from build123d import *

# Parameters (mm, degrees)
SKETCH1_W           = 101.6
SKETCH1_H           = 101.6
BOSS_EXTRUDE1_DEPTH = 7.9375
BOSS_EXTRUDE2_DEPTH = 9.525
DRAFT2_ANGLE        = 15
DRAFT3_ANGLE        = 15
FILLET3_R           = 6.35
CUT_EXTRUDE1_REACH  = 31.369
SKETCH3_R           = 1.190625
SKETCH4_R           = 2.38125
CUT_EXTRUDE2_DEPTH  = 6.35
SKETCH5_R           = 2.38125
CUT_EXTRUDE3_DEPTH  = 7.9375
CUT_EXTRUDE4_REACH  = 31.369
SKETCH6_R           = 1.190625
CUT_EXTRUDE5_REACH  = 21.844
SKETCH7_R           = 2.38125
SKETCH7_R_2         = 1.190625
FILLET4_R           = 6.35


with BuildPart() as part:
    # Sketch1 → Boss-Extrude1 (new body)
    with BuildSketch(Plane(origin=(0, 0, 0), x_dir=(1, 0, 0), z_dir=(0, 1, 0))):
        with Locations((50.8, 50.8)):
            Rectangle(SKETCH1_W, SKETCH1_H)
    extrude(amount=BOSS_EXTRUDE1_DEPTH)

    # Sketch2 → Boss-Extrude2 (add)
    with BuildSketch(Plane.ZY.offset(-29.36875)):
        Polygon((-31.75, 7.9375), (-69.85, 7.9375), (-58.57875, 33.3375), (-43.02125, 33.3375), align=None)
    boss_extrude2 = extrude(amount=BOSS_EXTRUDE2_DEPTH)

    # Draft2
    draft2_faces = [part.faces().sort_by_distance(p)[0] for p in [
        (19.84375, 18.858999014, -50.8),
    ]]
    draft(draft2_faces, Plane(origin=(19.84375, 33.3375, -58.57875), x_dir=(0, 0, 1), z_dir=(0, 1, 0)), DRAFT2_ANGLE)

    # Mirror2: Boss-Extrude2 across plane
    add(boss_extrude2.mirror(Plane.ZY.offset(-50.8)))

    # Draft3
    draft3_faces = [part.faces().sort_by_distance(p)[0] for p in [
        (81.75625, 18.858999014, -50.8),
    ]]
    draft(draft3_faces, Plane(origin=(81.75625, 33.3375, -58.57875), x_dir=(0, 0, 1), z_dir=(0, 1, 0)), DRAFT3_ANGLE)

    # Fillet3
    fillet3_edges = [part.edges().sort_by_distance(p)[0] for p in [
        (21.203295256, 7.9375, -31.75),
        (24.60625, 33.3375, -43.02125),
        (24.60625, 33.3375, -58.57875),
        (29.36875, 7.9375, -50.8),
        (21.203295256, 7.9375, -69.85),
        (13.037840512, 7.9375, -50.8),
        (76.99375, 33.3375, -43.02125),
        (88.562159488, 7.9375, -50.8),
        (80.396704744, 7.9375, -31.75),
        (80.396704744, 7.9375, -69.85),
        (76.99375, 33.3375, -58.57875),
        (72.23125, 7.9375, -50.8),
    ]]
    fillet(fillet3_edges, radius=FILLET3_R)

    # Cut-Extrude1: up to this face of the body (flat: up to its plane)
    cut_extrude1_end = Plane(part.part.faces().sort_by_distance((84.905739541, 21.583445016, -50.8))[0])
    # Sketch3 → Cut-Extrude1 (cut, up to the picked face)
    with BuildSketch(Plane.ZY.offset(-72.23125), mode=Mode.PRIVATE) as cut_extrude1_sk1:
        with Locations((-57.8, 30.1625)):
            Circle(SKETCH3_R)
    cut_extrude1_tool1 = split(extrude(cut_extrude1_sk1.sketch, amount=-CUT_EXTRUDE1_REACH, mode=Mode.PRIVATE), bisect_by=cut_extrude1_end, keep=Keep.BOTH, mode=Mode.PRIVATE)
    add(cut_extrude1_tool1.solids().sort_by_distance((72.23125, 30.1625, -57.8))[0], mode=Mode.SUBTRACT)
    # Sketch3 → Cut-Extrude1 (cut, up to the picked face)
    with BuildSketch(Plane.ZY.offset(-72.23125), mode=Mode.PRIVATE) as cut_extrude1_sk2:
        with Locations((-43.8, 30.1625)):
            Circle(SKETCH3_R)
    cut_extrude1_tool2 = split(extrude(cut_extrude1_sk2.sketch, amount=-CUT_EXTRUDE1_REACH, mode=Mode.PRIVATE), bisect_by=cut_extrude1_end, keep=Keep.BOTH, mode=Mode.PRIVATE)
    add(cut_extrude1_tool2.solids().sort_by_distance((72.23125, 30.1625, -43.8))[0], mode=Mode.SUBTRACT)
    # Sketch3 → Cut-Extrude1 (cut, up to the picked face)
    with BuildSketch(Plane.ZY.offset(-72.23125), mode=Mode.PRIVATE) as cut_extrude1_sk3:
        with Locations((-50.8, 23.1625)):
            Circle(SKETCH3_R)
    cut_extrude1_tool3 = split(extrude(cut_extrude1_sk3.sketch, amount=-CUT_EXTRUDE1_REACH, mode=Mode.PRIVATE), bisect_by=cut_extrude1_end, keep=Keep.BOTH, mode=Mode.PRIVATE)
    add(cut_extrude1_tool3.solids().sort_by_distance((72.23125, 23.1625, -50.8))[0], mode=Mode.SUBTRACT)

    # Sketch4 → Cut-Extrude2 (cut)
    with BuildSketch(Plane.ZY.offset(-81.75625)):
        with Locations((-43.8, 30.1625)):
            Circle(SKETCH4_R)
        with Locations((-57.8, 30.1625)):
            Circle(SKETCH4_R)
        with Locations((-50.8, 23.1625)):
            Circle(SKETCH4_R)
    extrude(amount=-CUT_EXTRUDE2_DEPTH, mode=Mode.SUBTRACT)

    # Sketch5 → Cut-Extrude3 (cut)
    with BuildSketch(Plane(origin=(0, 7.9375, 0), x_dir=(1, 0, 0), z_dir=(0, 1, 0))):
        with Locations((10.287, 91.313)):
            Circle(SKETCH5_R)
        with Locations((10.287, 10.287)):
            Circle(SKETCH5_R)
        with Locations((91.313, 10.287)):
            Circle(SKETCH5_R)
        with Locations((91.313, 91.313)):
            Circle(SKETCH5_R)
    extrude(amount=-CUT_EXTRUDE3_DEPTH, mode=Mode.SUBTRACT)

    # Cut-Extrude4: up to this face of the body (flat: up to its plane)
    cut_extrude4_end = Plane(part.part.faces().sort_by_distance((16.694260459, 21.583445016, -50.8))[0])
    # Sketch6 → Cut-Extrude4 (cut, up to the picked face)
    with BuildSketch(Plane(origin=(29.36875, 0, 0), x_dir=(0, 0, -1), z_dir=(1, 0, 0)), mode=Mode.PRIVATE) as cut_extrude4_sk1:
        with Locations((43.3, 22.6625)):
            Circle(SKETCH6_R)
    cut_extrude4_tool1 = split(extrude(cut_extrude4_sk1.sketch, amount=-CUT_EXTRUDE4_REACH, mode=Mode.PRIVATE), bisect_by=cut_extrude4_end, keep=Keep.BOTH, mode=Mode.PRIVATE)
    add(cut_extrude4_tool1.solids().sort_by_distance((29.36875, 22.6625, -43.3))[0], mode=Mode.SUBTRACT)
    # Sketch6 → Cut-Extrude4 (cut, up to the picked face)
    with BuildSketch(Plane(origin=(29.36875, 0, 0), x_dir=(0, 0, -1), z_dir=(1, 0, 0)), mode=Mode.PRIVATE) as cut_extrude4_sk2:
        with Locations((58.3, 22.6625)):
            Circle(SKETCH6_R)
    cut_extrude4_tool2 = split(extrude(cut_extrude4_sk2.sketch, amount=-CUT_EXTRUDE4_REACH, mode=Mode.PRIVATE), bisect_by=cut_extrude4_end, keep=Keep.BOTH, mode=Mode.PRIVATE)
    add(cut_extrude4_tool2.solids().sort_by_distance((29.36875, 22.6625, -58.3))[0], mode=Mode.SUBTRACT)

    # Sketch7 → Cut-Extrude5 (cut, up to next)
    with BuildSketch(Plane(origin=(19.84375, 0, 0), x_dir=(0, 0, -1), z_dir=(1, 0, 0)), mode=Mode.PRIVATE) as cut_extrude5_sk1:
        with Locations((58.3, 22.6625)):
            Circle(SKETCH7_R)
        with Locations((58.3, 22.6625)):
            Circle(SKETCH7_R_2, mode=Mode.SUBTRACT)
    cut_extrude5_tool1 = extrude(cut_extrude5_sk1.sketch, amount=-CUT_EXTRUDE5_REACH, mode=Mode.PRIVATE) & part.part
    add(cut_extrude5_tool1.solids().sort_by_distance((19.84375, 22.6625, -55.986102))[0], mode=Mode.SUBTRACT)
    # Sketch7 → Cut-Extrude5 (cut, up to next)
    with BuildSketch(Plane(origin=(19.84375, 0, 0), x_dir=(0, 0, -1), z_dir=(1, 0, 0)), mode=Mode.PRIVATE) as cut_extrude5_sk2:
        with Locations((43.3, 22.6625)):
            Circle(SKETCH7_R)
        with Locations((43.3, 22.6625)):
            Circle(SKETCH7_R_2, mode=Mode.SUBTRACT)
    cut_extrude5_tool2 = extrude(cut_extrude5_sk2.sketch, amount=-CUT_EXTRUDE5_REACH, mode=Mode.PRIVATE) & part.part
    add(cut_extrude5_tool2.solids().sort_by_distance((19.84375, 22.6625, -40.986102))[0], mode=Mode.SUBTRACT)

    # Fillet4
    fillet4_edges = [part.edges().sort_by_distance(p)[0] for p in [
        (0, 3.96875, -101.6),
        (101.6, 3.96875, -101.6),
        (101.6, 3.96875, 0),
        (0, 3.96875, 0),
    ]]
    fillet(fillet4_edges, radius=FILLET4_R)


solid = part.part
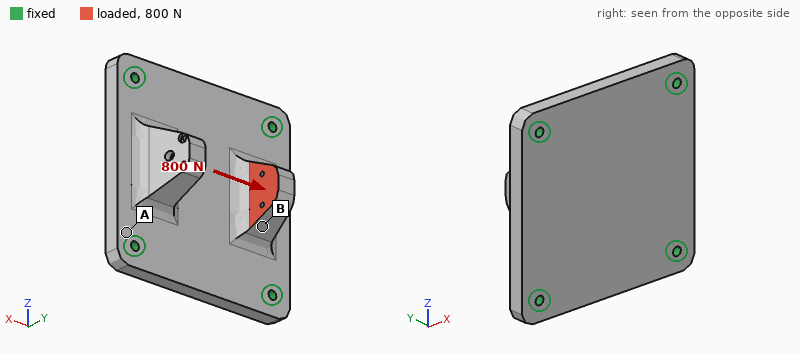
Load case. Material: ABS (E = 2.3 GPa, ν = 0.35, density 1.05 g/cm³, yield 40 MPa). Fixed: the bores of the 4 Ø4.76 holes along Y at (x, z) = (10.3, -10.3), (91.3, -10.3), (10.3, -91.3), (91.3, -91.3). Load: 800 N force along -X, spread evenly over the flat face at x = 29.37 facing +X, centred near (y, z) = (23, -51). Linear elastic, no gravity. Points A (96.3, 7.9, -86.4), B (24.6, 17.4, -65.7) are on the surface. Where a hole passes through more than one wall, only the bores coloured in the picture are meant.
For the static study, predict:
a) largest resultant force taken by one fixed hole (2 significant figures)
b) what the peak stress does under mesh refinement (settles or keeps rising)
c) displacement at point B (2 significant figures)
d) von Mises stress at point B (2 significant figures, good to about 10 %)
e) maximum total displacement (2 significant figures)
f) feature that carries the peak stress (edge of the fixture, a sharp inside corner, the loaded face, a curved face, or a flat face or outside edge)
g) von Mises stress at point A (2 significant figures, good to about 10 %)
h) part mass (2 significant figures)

270 N
keeps rising
0.27 mm
5.1 MPa
0.67 mm
edge of the fixture
1.5 MPa
110 g
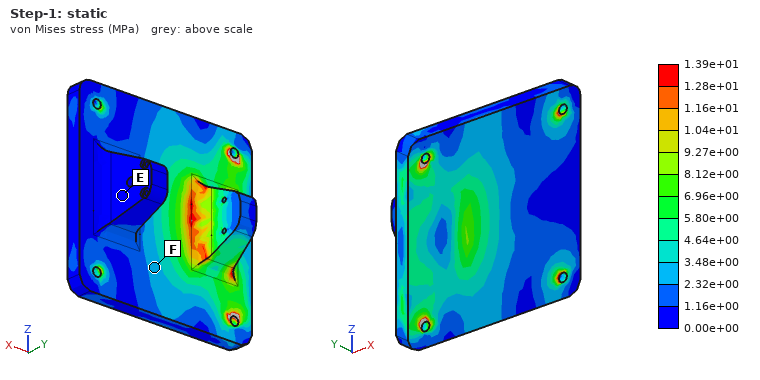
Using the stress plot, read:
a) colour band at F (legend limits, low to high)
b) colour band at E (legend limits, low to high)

2.32e+00 to 3.48e+00 MPa
0.00e+00 to 1.16e+00 MPa
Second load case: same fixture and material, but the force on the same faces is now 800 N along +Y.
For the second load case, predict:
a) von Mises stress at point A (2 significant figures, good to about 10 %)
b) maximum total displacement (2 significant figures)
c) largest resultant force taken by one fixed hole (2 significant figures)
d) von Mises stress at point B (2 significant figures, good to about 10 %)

2.8 MPa
0.53 mm
330 N
4.8 MPa
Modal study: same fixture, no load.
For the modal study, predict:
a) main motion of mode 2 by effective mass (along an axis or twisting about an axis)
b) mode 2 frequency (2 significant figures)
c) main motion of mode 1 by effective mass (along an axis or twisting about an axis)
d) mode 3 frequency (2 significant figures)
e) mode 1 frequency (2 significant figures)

twisting about Z
1800 Hz
along Y
1900 Hz
1100 Hz
